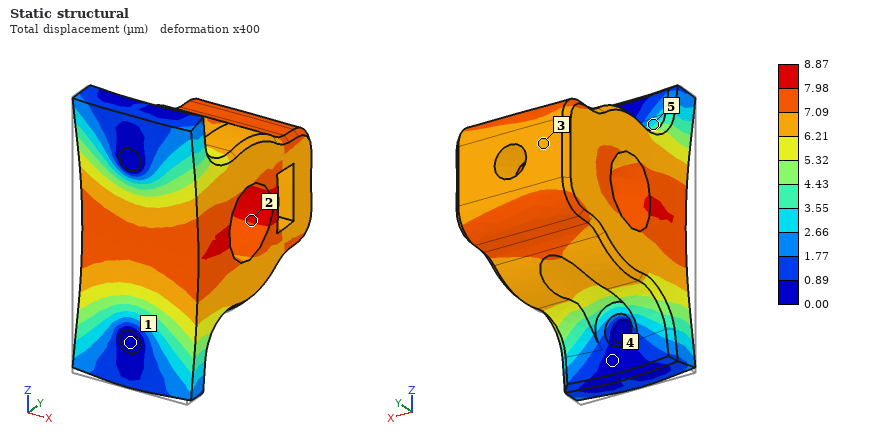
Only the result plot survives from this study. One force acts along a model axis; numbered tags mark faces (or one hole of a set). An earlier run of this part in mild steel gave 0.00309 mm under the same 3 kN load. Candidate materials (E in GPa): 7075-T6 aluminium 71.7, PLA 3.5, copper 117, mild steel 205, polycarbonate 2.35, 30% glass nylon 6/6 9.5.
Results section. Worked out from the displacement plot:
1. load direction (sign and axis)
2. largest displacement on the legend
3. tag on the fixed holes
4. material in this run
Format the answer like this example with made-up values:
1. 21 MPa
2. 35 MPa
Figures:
1. +Y
2. 8.87 µm
3. 1
4. 7075-T6 aluminium
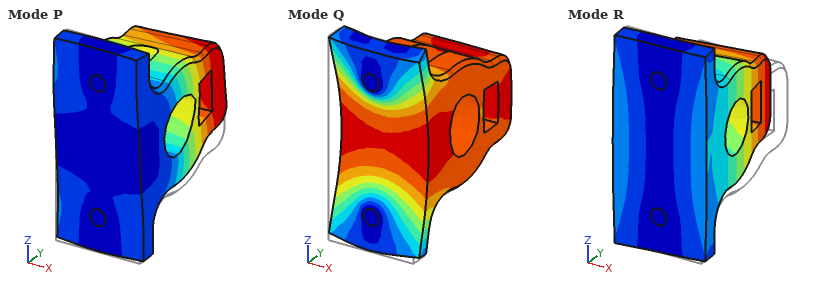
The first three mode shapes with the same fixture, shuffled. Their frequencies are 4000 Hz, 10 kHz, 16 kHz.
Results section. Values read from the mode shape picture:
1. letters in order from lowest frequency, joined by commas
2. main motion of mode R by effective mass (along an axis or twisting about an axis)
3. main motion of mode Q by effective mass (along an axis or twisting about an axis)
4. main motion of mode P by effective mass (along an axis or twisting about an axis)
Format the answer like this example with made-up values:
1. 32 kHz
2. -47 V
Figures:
1. R, P, Q
2. along X
3. along Y
4. along Z
